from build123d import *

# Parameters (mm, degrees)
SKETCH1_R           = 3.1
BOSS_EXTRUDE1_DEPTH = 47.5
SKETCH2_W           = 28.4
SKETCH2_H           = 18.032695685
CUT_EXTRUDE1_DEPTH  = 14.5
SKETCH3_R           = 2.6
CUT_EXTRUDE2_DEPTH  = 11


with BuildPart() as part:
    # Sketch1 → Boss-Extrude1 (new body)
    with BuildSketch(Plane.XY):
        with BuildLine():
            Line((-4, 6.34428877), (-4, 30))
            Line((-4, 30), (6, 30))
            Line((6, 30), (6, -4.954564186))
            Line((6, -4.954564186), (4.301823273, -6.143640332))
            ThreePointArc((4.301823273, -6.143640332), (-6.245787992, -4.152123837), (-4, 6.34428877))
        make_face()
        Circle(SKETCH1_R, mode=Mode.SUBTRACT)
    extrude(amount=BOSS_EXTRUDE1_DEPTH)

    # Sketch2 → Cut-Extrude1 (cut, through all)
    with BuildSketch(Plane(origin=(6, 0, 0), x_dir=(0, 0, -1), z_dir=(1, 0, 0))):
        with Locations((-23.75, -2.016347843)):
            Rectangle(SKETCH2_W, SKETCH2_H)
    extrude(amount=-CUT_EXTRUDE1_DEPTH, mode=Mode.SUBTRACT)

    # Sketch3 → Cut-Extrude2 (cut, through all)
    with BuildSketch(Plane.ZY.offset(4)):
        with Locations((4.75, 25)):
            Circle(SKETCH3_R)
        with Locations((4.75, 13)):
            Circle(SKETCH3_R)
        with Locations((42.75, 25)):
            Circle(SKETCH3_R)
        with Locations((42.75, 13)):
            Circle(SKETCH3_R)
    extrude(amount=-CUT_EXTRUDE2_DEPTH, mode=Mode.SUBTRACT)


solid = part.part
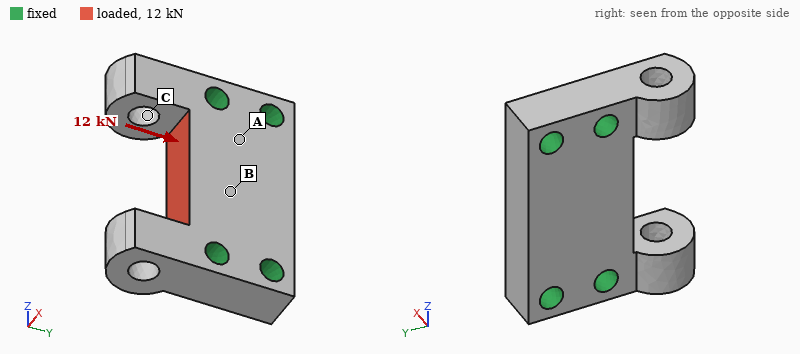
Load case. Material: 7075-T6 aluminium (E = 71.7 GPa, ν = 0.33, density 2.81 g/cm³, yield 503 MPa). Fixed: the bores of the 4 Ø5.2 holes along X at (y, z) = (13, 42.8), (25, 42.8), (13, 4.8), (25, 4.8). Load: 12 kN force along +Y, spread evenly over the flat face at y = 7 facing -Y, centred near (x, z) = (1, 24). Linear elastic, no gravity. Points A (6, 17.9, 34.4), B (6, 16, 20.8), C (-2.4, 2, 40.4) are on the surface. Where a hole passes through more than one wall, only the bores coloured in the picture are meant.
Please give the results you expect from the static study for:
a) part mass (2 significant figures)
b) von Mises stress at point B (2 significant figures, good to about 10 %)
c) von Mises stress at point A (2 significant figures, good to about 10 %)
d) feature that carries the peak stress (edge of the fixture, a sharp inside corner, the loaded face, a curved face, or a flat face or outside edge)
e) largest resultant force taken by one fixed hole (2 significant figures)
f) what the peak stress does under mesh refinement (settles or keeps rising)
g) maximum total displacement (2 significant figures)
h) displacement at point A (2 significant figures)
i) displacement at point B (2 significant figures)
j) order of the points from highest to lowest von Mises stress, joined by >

36 g
30 MPa
53 MPa
edge of the fixture
3.6 kN
keeps rising
19 µm
7.7 µm
14 µm
A > B > C
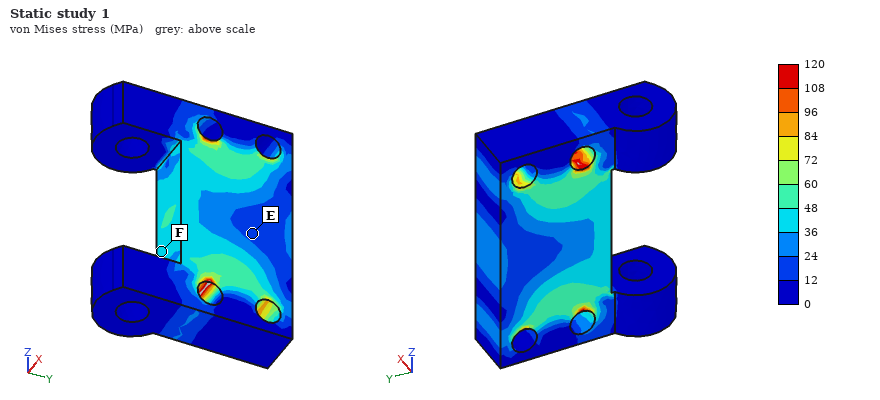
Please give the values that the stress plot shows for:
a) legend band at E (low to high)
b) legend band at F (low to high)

12 to 24 MPa
36 to 48 MPa
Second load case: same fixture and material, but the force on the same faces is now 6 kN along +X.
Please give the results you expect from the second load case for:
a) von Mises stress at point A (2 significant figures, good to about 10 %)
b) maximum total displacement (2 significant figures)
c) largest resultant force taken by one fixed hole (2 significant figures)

49 MPa
41 µm
3.2 kN
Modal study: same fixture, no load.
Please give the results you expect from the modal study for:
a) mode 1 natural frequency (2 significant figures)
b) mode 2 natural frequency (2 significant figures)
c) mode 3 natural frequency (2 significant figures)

18 kHz
18 kHz
19 kHz
